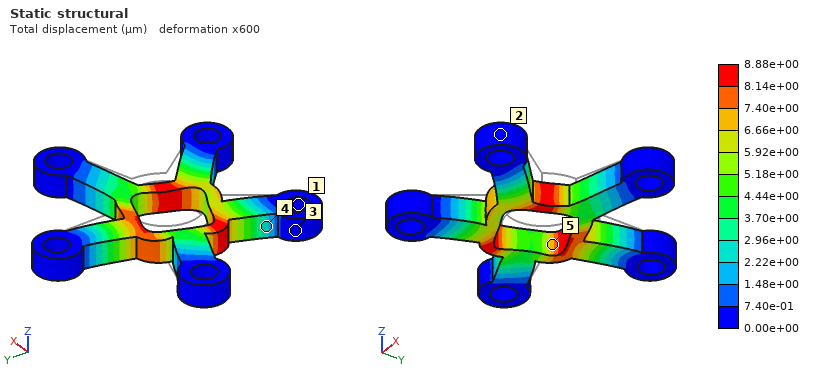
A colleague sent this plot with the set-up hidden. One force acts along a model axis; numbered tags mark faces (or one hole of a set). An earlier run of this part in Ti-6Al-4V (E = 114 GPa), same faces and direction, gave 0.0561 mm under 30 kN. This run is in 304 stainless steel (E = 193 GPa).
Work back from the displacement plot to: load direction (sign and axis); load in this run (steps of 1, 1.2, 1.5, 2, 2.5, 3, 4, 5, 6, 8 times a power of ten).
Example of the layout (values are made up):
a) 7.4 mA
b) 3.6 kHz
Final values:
a) -X
b) 8 kN
